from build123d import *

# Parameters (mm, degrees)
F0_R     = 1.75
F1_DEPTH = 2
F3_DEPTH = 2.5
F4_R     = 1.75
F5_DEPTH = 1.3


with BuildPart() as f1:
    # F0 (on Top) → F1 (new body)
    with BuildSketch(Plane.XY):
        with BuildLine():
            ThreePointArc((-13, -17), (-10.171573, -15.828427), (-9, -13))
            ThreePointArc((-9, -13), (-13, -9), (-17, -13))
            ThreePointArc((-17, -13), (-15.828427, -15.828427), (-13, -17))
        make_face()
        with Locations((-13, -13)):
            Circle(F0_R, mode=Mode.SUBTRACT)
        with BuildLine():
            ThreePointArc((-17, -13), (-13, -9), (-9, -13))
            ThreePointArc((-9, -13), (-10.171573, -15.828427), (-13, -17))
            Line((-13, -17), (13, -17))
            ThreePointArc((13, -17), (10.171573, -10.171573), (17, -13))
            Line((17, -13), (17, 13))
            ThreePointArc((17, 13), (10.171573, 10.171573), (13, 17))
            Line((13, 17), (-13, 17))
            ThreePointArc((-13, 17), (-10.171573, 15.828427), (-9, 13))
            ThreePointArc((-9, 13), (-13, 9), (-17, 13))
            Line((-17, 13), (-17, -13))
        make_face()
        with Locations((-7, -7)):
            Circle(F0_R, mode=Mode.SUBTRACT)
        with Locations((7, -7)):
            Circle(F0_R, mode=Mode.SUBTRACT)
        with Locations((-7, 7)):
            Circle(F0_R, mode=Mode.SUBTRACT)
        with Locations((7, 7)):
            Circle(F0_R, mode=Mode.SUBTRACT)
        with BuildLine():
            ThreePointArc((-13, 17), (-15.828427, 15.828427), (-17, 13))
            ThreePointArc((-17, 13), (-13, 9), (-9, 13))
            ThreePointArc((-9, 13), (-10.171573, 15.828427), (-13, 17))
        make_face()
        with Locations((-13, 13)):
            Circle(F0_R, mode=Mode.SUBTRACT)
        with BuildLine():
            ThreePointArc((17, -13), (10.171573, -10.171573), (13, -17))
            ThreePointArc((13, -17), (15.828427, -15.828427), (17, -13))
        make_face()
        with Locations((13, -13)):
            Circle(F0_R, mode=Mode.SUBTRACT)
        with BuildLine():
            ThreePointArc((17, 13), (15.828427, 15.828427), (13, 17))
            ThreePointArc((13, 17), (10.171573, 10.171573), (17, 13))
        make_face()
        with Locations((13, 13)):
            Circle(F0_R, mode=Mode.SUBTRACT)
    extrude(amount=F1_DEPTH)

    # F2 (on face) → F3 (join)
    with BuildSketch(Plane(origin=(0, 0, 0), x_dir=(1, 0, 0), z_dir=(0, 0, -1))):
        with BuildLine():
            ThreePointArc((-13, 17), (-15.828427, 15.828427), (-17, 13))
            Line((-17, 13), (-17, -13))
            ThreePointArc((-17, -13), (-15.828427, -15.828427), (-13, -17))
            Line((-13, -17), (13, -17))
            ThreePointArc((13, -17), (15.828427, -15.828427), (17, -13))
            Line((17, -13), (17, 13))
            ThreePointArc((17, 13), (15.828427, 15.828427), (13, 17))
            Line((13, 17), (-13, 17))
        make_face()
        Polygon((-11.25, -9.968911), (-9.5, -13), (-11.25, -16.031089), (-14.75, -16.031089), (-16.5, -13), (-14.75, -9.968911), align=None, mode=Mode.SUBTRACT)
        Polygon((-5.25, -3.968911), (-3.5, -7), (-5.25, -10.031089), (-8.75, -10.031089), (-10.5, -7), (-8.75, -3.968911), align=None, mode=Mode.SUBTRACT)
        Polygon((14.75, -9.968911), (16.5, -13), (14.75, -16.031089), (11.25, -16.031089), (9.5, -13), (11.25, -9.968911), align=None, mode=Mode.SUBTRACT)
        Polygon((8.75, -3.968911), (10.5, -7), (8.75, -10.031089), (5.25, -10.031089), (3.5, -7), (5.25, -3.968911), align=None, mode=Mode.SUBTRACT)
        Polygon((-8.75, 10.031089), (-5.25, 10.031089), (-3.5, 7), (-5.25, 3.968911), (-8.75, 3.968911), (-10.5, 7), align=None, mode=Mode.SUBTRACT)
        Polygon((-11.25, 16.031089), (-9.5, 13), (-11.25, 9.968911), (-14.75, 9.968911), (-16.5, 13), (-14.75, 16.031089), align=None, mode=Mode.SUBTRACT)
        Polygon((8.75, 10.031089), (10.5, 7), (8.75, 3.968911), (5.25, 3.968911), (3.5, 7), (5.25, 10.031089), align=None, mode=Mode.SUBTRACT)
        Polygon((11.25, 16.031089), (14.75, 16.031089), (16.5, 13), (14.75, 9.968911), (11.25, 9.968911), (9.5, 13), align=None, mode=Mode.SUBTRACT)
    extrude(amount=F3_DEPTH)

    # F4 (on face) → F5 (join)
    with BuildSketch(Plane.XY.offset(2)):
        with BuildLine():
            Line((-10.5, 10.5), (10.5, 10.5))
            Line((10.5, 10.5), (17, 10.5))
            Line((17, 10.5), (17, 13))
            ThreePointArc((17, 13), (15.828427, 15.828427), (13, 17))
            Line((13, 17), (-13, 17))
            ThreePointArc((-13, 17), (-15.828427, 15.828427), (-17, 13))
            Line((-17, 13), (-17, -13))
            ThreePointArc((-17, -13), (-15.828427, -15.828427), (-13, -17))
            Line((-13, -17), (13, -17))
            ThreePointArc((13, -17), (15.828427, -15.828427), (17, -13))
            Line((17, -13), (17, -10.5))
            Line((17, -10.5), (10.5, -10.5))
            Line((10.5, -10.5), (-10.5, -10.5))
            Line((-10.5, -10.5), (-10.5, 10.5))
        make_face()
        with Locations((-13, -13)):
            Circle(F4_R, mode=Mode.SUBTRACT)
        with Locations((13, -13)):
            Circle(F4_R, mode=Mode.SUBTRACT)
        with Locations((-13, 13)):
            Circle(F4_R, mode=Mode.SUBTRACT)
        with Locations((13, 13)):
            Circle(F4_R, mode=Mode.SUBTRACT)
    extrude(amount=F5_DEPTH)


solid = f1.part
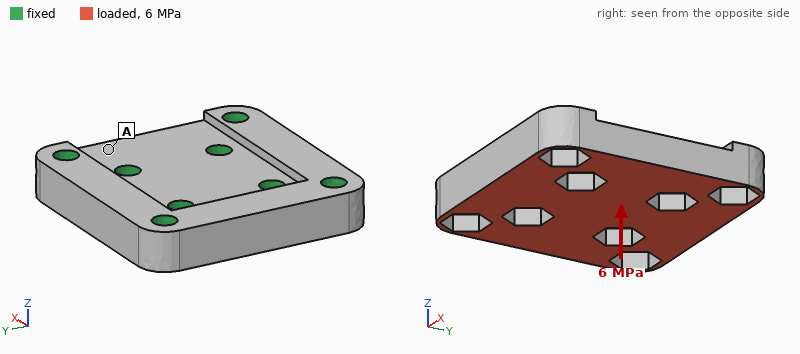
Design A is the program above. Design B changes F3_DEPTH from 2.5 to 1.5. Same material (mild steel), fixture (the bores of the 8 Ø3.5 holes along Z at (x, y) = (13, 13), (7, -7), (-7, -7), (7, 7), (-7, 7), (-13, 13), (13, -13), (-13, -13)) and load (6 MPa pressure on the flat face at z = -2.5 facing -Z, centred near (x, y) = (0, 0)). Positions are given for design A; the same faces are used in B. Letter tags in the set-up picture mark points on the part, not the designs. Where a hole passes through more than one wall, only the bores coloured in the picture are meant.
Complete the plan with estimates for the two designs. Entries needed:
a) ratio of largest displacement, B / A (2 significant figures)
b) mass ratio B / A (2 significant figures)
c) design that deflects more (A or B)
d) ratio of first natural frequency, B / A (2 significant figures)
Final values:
1.7
0.82
B
0.94
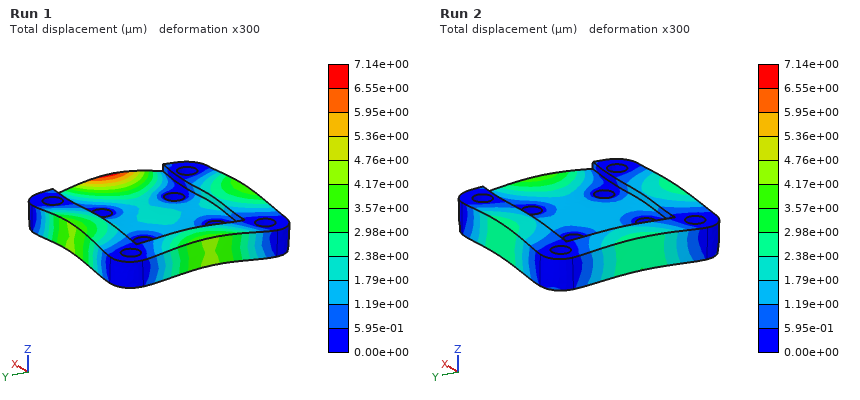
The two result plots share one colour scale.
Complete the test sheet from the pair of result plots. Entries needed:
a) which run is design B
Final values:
Run 1
